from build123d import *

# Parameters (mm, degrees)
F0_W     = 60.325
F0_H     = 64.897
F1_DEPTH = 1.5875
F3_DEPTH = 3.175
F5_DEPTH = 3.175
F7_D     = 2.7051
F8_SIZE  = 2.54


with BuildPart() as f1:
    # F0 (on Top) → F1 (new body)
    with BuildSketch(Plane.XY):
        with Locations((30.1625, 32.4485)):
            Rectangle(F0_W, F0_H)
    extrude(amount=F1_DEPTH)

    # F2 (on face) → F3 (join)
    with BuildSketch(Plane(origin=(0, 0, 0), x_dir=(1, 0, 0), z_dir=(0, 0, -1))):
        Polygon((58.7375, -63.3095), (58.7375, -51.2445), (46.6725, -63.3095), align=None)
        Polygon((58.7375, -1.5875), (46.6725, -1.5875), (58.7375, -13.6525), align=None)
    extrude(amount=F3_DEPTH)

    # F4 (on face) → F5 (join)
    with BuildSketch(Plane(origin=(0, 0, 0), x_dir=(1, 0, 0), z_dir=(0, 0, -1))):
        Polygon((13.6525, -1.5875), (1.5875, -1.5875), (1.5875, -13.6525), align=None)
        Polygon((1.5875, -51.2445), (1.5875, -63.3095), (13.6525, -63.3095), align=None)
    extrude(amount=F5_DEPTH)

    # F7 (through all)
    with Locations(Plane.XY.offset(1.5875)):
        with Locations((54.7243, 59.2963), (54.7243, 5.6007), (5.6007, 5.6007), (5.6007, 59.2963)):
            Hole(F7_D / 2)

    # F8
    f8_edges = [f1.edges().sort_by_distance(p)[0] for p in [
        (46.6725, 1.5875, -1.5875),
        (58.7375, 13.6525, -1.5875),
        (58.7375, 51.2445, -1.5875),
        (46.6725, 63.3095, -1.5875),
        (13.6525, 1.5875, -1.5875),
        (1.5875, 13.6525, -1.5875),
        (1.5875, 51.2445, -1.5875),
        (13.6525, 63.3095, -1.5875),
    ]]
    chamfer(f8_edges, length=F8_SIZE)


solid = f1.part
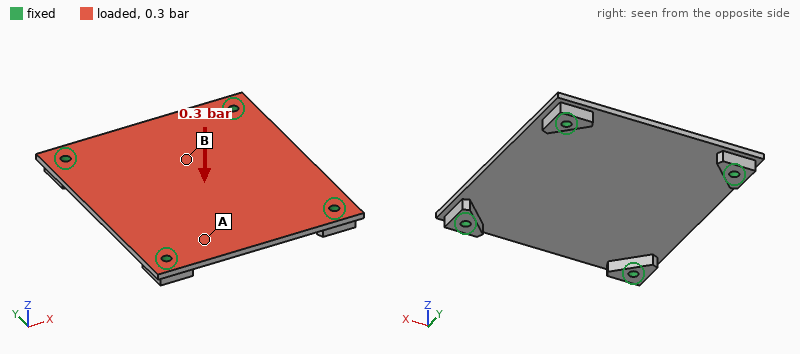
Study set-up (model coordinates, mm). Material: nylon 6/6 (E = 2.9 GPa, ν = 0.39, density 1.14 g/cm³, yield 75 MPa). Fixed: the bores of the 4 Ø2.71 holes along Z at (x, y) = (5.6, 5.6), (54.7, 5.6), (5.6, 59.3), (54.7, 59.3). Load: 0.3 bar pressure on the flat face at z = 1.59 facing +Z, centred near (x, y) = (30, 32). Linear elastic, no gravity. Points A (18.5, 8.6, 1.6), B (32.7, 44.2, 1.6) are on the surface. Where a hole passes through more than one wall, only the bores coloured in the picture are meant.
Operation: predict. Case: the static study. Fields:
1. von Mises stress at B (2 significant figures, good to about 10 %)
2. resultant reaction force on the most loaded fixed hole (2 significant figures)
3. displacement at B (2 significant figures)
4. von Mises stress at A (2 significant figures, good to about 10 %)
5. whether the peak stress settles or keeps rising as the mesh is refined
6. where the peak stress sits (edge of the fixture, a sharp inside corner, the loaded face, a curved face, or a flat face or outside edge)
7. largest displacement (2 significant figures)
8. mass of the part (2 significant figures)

7.9 MPa
34 N
0.83 mm
3.8 MPa
keeps rising
edge of the fixture
1.0 mm
7.9 g
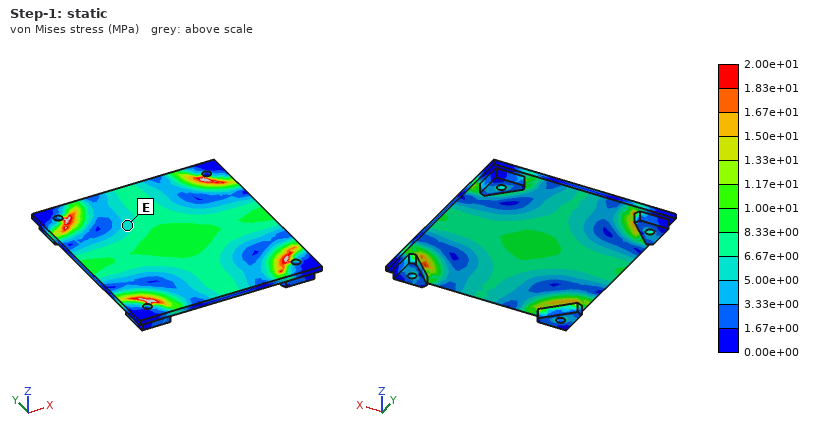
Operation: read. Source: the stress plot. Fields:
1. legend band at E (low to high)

5.00e+00 to 6.67e+00 MPa
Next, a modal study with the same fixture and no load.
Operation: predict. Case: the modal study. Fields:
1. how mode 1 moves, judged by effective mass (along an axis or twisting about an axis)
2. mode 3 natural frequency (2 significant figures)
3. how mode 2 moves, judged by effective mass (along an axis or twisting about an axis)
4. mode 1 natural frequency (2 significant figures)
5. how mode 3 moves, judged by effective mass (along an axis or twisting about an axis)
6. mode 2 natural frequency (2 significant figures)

along Z
1500 Hz
twisting about Y
800 Hz
twisting about X
1300 Hz
